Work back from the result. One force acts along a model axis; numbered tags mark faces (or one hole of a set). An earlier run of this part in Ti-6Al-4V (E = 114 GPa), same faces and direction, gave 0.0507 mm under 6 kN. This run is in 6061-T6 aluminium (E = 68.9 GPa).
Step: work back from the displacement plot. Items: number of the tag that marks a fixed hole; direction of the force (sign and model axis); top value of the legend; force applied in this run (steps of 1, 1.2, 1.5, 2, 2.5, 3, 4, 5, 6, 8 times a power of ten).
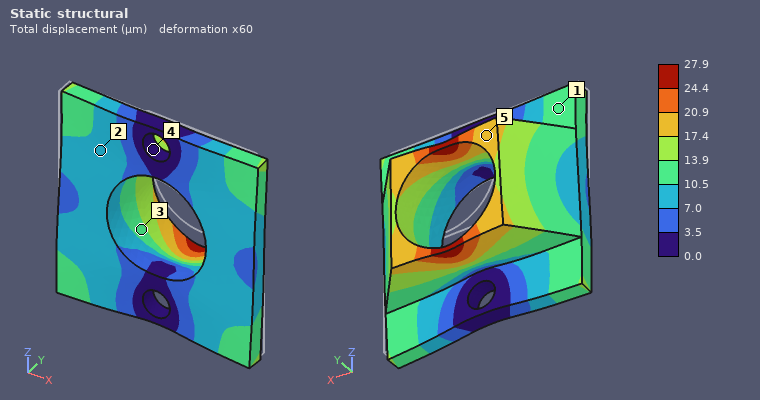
4
-Z
27.9 µm
2 kN
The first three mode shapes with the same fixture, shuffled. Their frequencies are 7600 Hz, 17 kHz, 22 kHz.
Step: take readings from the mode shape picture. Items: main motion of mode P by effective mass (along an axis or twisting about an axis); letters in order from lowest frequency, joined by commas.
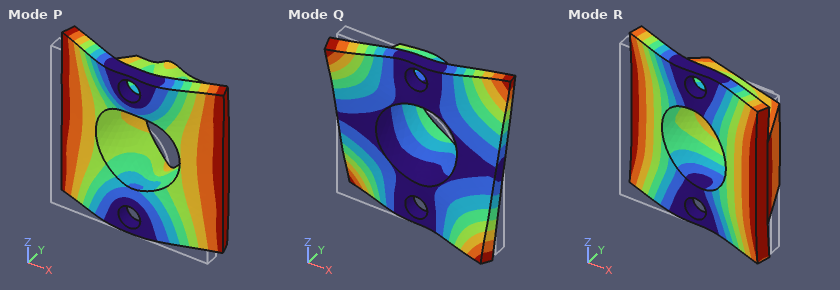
along Y
R, P, Q
